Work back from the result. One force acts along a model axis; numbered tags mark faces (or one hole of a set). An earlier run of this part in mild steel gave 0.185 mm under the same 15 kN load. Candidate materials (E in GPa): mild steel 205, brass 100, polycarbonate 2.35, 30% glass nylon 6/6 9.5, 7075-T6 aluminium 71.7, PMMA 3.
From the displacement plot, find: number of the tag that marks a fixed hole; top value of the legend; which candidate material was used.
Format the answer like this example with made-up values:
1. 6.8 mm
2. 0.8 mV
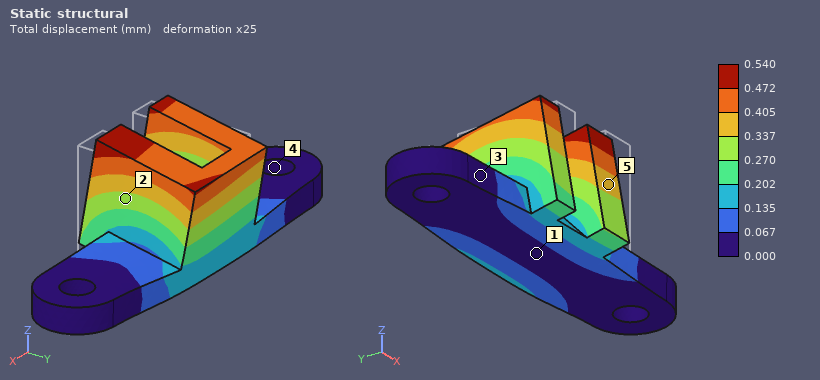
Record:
1. 4
2. 0.540 mm
3. 7075-T6 aluminium
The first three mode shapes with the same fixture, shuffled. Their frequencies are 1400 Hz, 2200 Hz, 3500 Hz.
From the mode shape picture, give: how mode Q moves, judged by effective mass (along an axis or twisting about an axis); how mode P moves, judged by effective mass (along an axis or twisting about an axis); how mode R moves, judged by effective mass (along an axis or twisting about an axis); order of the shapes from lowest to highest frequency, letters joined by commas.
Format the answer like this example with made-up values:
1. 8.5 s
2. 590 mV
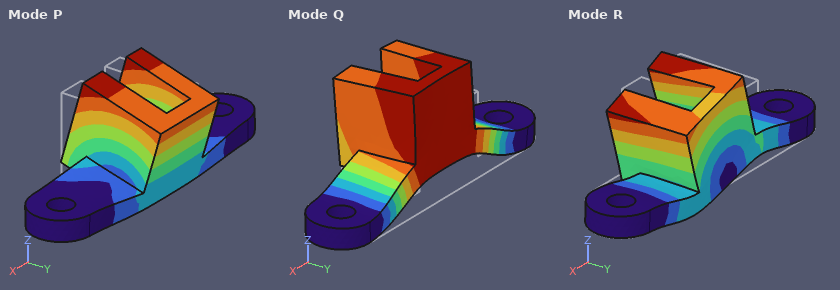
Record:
1. along Z
2. along Y
3. along X
4. P, Q, R
